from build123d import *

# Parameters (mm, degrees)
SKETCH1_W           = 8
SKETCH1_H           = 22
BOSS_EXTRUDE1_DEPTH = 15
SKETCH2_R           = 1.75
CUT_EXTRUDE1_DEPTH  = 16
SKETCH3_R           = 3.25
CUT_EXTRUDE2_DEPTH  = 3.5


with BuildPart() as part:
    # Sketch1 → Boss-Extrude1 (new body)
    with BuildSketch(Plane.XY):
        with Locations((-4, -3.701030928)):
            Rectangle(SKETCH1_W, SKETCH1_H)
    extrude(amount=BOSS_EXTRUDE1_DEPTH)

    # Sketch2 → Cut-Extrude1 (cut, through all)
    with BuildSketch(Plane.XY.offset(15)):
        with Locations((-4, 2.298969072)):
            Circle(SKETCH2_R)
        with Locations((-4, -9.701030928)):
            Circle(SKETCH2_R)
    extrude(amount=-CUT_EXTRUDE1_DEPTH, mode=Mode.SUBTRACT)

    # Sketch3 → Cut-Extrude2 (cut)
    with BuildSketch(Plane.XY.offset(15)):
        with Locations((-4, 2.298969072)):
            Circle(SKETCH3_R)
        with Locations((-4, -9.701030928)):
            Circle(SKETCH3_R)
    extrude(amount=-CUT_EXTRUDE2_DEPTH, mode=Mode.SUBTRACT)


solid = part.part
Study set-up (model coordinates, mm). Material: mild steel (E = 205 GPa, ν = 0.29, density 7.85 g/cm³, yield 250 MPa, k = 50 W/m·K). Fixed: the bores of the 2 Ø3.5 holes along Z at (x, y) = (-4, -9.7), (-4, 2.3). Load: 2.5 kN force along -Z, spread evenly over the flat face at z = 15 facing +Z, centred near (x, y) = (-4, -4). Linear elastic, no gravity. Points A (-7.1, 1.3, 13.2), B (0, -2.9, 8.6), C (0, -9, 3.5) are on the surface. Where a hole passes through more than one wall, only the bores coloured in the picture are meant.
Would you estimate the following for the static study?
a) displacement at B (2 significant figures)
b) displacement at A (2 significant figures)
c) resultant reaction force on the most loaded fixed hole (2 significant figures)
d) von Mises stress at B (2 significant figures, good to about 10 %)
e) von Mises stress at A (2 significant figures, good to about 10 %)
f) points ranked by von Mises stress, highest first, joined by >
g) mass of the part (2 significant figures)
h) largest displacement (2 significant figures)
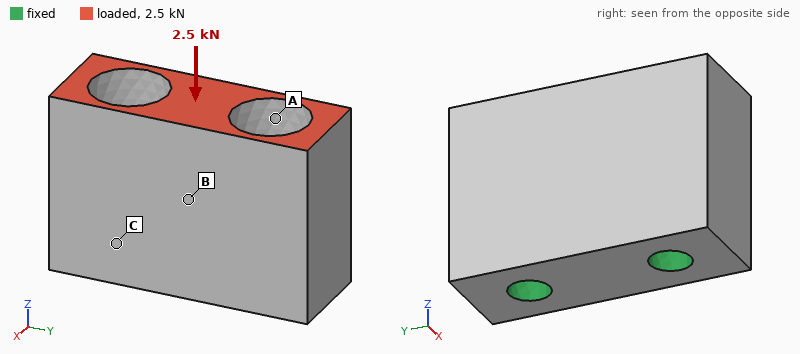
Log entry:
0.42 µm
0.68 µm
1.3 kN
13 MPa
27 MPa
A > B > C
17 g
1.1 µm
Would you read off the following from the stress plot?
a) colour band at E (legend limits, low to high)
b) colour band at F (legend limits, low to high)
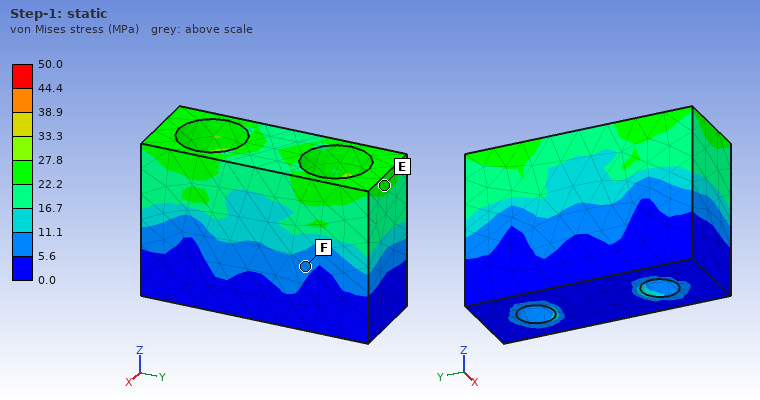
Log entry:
22.2 to 27.8 MPa
5.6 to 11.1 MPa
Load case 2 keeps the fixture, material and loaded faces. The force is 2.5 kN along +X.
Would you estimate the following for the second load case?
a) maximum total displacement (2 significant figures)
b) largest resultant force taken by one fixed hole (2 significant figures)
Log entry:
7.5 µm
1.3 kN
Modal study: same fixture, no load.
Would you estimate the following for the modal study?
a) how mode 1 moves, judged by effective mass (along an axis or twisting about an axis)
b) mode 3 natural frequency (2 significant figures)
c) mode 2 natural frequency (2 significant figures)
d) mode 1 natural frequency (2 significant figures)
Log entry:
along X
86 kHz
86 kHz
77 kHz
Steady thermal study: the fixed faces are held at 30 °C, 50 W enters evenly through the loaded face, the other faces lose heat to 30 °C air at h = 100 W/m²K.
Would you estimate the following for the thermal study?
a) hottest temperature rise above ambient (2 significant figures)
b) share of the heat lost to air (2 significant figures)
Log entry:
57 K
3.6 %
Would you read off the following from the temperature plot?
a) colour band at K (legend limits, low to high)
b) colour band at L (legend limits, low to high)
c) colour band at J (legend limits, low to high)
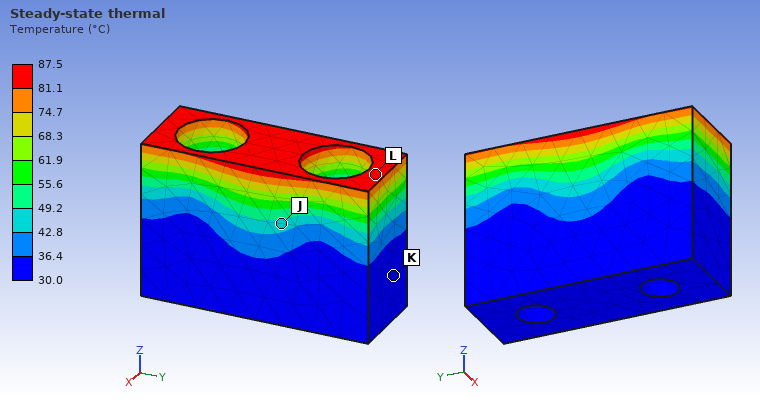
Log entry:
30.0 to 36.4 °C
81.1 to 87.5 °C
42.8 to 49.2 °C
